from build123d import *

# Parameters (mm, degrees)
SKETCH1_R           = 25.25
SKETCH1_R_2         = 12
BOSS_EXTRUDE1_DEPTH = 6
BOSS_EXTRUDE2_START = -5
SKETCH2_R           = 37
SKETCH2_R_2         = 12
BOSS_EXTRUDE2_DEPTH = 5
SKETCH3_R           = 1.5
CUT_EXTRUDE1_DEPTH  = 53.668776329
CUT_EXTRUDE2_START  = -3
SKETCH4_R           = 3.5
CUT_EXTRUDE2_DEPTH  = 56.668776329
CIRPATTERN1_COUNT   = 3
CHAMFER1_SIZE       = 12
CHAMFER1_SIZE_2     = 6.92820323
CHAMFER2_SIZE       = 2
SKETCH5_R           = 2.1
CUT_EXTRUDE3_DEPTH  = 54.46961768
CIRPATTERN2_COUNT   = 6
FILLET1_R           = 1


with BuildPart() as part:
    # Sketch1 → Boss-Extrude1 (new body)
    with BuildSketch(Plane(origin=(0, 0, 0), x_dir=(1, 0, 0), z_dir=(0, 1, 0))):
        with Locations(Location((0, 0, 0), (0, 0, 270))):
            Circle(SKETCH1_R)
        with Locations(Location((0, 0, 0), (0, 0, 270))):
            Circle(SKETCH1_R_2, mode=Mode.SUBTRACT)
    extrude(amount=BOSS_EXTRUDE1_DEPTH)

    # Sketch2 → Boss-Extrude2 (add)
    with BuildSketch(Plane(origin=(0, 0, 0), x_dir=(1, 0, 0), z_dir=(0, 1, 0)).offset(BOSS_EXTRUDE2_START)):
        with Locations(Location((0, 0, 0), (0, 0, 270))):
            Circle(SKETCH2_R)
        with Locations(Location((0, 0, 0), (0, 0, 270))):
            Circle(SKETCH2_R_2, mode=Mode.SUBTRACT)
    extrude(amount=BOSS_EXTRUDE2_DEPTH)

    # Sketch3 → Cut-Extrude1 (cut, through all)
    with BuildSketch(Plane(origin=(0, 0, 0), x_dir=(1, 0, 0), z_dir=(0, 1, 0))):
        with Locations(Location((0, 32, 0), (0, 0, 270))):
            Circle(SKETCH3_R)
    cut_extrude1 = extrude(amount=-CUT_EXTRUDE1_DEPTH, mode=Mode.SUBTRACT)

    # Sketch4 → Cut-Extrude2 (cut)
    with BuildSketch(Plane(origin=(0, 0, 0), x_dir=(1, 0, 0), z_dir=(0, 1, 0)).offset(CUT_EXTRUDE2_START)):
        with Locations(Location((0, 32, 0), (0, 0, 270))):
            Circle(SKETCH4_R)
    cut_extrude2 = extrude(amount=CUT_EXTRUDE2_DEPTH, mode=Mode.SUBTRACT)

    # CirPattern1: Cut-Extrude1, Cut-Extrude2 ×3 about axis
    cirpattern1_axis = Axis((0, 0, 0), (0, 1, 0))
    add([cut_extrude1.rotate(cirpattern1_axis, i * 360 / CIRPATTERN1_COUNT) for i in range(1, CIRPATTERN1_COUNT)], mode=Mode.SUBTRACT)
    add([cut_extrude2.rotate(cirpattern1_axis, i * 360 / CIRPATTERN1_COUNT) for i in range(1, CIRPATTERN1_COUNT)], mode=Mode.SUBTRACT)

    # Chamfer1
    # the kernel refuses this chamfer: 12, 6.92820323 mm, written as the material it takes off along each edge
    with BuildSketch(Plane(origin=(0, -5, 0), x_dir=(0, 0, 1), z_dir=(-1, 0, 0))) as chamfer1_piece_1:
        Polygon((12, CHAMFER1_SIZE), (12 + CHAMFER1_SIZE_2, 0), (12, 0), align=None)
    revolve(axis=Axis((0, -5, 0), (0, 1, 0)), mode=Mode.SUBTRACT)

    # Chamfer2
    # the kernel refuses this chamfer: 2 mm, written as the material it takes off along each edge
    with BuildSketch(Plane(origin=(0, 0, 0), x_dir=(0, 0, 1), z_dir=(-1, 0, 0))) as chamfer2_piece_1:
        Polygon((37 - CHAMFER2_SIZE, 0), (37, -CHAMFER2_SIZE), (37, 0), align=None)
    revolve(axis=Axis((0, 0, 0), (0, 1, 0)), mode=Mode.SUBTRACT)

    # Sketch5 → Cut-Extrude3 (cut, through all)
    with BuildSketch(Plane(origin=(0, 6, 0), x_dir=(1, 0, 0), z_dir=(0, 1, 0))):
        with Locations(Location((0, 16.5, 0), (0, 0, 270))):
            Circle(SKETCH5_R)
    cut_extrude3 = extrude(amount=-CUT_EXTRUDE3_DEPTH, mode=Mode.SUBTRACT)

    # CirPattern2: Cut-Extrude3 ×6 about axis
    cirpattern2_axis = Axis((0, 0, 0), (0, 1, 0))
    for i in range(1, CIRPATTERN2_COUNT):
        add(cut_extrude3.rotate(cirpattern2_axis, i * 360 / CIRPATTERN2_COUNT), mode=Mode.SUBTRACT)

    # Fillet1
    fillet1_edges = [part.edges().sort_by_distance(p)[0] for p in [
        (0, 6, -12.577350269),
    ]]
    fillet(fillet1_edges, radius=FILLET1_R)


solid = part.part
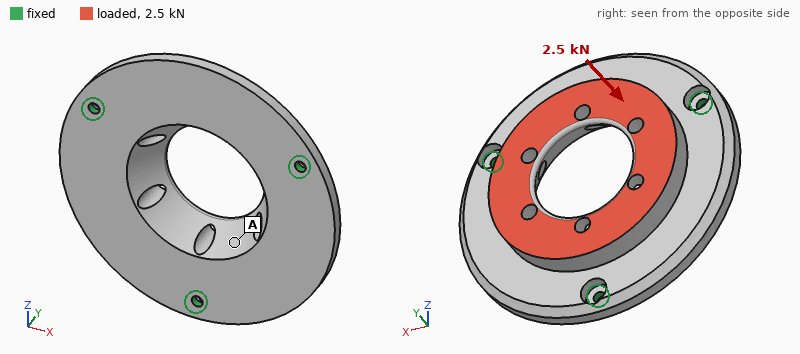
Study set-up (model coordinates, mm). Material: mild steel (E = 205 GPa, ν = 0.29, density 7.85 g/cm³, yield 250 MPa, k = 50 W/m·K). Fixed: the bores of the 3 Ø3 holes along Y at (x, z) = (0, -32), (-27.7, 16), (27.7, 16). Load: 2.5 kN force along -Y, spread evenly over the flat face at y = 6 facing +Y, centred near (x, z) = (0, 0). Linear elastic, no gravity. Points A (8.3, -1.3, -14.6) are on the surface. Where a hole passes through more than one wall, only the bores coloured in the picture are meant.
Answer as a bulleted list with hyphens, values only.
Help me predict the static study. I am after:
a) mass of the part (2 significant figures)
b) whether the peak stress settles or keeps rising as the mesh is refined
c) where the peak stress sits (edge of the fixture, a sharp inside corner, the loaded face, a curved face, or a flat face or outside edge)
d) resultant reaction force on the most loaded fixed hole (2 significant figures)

- 180 g
- keeps rising
- edge of the fixture
- 1.2 kN
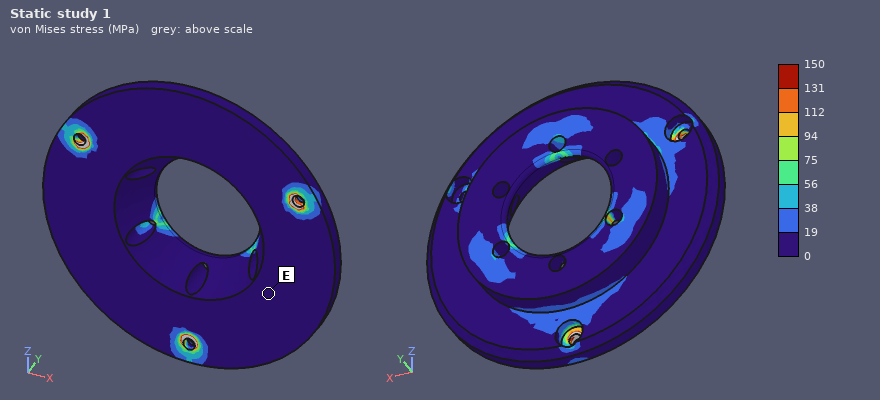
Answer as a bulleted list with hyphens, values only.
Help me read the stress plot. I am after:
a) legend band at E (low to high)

- 0 to 19 MPa
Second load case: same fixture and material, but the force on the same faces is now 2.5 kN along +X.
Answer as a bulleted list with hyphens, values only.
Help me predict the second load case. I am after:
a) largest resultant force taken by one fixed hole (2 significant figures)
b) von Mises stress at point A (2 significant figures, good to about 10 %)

- 1.0 kN
- 11 MPa
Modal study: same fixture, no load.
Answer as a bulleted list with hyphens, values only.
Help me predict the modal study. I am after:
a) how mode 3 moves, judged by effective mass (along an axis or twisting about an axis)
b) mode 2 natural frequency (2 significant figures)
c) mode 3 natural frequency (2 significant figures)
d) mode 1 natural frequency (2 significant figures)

- along Y
- 5600 Hz
- 6800 Hz
- 5600 Hz
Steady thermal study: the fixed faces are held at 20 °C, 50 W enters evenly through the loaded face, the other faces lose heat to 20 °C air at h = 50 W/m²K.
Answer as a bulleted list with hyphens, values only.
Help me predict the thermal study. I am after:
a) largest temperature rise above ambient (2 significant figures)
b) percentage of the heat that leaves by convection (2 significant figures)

- 46 K
- 32 %
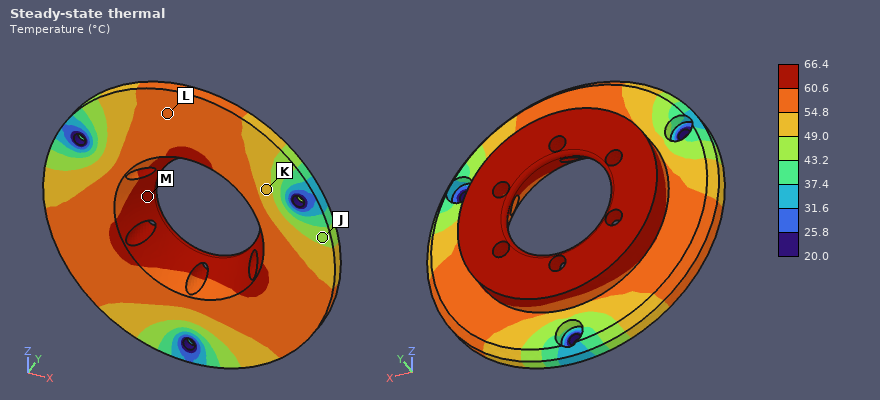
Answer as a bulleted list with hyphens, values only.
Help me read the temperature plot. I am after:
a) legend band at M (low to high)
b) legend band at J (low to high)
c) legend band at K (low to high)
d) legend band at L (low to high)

- 60.6 to 66.4 °C
- 43.2 to 49.0 °C
- 49.0 to 54.8 °C
- 54.8 to 60.6 °C
